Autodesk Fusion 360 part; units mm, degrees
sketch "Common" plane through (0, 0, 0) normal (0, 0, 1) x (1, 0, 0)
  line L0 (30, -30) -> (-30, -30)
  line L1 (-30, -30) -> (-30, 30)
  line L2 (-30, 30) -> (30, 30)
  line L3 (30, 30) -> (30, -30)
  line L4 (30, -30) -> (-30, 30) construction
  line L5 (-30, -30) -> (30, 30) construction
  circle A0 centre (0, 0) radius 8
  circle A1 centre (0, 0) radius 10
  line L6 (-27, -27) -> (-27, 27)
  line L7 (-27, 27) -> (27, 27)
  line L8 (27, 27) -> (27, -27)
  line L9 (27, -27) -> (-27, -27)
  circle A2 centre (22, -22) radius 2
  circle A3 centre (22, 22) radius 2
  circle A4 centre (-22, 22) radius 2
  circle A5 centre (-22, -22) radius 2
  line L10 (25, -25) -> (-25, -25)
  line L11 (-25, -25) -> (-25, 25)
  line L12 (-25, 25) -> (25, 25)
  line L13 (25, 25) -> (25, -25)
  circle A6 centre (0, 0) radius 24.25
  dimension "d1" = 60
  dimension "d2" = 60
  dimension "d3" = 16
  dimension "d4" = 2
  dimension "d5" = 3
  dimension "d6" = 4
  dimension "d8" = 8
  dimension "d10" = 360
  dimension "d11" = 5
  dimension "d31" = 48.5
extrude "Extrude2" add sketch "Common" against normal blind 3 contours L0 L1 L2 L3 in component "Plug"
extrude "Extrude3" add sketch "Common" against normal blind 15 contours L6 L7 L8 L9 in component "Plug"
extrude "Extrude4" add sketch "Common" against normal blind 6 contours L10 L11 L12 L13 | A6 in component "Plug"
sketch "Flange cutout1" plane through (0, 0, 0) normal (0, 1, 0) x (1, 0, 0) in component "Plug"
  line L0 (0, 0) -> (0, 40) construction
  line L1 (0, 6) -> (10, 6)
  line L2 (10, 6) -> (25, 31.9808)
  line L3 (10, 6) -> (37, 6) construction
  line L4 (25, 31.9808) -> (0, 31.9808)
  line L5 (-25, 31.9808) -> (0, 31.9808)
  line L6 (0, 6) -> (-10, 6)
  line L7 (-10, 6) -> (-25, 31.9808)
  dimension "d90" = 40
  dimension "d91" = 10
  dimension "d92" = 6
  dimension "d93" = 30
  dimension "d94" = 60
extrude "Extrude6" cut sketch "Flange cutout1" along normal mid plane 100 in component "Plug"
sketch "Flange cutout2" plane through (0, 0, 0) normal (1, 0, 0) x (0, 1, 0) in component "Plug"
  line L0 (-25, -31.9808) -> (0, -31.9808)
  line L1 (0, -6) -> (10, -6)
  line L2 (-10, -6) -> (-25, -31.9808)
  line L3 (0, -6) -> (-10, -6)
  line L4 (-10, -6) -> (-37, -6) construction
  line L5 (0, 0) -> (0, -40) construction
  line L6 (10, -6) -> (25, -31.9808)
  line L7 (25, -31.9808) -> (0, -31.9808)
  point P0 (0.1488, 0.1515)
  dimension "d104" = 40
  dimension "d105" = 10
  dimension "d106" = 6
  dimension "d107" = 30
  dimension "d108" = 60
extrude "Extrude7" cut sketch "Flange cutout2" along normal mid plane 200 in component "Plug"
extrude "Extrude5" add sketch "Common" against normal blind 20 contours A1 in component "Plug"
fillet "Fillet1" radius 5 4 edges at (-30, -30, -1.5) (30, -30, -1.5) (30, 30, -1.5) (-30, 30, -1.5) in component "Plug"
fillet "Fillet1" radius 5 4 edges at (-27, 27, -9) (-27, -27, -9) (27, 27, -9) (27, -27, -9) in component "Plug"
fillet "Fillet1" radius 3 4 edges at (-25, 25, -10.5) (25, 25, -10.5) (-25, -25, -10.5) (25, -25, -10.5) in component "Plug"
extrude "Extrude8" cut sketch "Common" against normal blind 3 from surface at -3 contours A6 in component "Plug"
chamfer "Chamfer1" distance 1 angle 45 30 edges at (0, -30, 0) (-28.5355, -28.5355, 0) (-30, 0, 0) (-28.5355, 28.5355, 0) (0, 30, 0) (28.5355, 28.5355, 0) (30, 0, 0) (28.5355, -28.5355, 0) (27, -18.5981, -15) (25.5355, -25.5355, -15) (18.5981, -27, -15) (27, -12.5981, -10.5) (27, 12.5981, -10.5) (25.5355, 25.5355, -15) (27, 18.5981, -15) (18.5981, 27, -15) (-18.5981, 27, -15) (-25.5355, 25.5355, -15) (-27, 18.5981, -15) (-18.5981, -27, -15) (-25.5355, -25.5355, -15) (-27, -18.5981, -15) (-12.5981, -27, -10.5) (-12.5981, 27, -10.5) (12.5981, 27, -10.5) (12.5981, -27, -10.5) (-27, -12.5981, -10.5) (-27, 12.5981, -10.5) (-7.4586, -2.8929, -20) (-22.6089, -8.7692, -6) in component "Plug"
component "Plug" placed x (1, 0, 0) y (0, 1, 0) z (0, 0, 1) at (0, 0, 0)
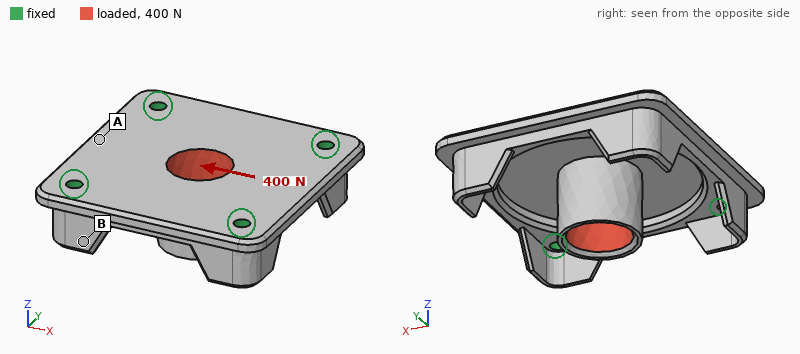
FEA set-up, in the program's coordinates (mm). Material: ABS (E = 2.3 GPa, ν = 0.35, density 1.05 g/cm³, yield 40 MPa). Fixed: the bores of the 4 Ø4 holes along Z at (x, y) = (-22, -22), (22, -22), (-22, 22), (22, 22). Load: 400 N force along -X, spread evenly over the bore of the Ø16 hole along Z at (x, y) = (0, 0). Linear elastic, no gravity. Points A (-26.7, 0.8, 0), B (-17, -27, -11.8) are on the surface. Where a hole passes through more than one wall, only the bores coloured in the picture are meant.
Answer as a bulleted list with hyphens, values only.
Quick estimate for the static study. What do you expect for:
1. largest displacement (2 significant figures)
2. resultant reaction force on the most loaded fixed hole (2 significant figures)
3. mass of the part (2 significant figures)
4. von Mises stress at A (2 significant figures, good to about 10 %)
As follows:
- 0.56 mm
- 110 N
- 17 g
- 4.1 MPa
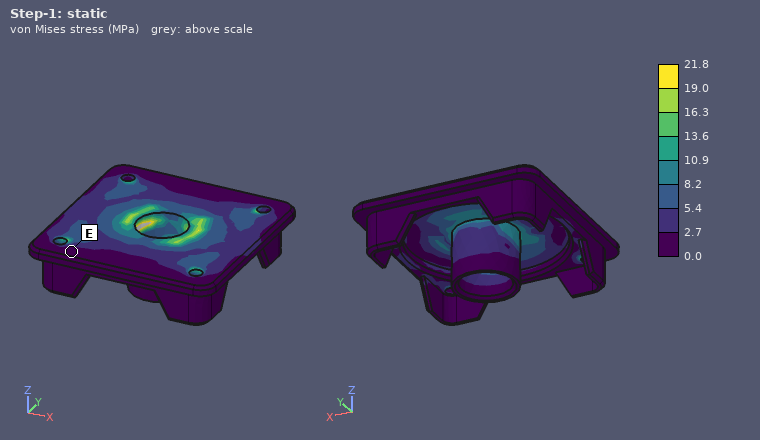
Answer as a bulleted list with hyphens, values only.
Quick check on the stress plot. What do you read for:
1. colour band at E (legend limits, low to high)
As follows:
- 0.0 to 2.7 MPa
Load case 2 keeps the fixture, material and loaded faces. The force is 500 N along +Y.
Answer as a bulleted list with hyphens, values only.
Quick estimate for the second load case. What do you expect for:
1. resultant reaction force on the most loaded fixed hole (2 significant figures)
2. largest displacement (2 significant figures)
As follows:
- 140 N
- 0.70 mm
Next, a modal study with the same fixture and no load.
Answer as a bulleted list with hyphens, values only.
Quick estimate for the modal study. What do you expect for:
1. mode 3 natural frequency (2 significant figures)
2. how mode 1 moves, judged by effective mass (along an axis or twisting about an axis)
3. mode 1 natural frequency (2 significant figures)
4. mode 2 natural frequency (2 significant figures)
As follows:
- 2700 Hz
- along Z
- 2200 Hz
- 2700 Hz
